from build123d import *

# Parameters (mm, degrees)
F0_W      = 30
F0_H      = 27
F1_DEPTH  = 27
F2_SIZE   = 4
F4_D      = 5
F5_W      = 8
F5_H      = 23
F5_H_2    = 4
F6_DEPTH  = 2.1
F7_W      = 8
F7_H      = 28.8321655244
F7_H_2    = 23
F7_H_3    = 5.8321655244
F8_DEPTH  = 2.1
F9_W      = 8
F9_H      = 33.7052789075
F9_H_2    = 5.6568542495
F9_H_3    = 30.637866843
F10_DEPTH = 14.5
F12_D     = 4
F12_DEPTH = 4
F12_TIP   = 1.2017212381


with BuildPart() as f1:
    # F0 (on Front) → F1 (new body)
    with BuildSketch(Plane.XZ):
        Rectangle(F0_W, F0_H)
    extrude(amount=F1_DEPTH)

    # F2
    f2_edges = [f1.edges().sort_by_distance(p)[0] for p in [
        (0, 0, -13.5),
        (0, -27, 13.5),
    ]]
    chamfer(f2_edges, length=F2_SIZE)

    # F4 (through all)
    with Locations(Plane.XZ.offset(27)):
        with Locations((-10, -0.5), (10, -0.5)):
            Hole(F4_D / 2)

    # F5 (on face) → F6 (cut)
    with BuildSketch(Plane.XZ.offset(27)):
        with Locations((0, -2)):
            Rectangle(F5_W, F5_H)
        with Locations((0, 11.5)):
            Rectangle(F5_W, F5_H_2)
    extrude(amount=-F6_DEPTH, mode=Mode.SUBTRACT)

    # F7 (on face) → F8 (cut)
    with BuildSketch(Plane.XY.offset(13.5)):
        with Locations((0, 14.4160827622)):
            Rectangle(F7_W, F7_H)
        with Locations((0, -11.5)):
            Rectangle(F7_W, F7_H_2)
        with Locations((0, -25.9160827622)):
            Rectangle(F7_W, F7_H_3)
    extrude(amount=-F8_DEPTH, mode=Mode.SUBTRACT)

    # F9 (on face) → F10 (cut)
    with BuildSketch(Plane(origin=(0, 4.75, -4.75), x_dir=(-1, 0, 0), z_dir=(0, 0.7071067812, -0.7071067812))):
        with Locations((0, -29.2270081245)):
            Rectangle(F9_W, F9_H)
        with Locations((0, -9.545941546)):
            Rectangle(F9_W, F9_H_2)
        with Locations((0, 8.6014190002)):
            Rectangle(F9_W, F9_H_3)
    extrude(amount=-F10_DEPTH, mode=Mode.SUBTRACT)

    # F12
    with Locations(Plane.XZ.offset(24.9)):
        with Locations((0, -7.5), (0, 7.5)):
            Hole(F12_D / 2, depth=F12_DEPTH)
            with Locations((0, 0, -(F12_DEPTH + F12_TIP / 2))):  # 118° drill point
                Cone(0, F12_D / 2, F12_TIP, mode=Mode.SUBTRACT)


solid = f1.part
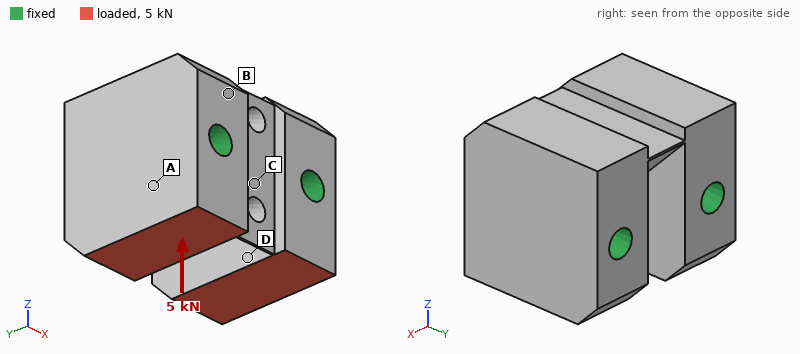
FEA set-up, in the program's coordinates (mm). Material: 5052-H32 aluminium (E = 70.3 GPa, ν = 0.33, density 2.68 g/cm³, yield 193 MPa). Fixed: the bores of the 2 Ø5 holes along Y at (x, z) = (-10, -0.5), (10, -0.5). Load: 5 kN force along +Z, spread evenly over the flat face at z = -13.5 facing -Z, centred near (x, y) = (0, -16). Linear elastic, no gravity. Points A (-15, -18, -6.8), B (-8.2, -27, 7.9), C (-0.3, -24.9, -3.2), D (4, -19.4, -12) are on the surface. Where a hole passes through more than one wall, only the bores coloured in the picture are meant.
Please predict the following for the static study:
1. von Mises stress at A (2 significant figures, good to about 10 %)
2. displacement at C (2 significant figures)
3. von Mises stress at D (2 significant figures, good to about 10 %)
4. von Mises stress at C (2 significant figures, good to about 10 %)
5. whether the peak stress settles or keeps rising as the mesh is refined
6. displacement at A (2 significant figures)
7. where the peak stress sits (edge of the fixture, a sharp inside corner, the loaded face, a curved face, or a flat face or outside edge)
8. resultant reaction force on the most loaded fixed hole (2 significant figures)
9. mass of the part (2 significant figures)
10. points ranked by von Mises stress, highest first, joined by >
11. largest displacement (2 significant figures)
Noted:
7.7 MPa
0.66 µm
9.9 MPa
2.7 MPa
keeps rising
0.89 µm
edge of the fixture
2.5 kN
46 g
D > A > C > B
2.1 µm
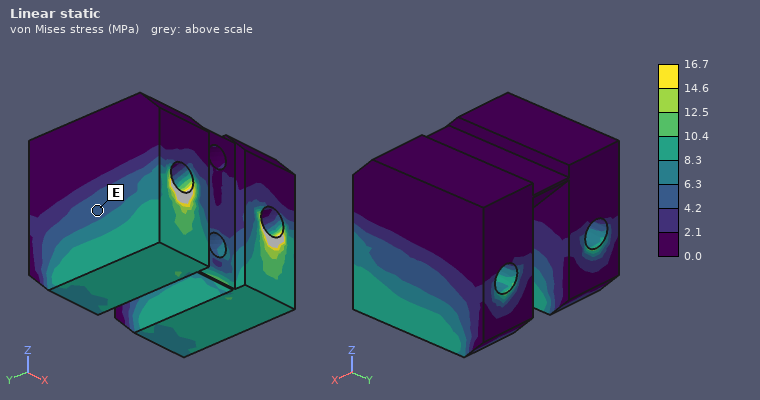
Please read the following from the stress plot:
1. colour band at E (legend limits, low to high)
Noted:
4.2 to 6.3 MPa
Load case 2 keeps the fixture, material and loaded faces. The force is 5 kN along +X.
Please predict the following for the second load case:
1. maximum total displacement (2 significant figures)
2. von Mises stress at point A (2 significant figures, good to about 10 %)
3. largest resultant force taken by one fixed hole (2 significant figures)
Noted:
13 µm
26 MPa
3.0 kN
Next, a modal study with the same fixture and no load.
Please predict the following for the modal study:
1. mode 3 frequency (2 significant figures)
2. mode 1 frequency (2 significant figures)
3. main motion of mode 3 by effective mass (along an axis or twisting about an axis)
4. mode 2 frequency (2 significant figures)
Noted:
48 kHz
43 kHz
along X
44 kHz
